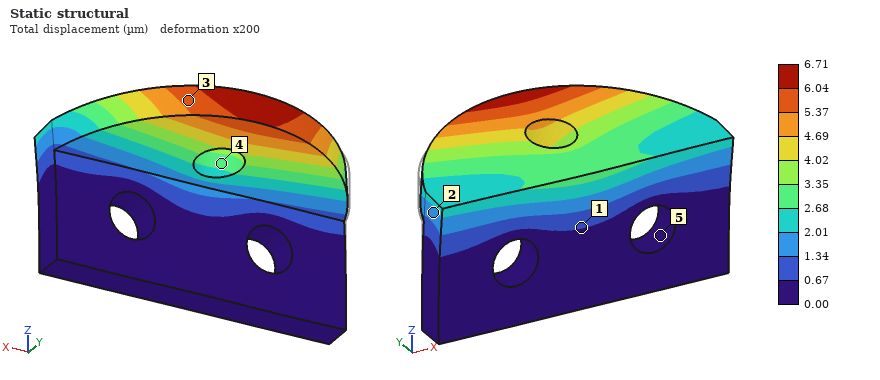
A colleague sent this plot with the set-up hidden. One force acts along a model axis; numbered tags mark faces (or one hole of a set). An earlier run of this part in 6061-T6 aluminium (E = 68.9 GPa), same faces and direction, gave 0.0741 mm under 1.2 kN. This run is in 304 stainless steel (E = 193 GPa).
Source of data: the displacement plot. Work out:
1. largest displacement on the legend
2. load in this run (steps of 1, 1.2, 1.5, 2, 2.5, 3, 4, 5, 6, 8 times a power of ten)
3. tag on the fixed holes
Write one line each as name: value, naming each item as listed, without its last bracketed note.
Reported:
largest displacement on the legend: 6.71 µm
load in this run: 300 N
tag on the fixed holes: 5
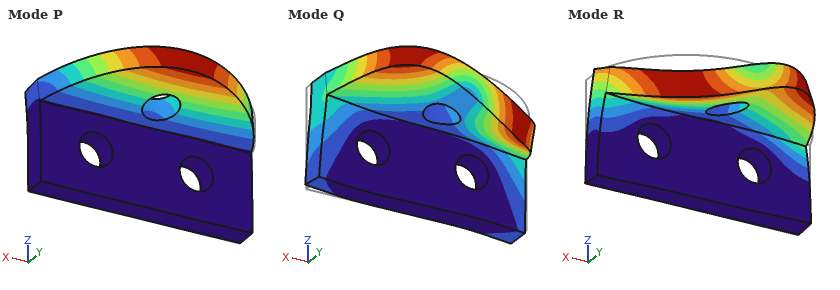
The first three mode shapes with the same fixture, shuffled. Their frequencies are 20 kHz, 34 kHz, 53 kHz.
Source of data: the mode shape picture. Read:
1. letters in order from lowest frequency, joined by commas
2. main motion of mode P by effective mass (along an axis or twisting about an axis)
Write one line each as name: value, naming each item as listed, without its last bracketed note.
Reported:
letters in order from lowest frequency, joined by commas: P, R, Q
main motion of mode P by effective mass: along Z
